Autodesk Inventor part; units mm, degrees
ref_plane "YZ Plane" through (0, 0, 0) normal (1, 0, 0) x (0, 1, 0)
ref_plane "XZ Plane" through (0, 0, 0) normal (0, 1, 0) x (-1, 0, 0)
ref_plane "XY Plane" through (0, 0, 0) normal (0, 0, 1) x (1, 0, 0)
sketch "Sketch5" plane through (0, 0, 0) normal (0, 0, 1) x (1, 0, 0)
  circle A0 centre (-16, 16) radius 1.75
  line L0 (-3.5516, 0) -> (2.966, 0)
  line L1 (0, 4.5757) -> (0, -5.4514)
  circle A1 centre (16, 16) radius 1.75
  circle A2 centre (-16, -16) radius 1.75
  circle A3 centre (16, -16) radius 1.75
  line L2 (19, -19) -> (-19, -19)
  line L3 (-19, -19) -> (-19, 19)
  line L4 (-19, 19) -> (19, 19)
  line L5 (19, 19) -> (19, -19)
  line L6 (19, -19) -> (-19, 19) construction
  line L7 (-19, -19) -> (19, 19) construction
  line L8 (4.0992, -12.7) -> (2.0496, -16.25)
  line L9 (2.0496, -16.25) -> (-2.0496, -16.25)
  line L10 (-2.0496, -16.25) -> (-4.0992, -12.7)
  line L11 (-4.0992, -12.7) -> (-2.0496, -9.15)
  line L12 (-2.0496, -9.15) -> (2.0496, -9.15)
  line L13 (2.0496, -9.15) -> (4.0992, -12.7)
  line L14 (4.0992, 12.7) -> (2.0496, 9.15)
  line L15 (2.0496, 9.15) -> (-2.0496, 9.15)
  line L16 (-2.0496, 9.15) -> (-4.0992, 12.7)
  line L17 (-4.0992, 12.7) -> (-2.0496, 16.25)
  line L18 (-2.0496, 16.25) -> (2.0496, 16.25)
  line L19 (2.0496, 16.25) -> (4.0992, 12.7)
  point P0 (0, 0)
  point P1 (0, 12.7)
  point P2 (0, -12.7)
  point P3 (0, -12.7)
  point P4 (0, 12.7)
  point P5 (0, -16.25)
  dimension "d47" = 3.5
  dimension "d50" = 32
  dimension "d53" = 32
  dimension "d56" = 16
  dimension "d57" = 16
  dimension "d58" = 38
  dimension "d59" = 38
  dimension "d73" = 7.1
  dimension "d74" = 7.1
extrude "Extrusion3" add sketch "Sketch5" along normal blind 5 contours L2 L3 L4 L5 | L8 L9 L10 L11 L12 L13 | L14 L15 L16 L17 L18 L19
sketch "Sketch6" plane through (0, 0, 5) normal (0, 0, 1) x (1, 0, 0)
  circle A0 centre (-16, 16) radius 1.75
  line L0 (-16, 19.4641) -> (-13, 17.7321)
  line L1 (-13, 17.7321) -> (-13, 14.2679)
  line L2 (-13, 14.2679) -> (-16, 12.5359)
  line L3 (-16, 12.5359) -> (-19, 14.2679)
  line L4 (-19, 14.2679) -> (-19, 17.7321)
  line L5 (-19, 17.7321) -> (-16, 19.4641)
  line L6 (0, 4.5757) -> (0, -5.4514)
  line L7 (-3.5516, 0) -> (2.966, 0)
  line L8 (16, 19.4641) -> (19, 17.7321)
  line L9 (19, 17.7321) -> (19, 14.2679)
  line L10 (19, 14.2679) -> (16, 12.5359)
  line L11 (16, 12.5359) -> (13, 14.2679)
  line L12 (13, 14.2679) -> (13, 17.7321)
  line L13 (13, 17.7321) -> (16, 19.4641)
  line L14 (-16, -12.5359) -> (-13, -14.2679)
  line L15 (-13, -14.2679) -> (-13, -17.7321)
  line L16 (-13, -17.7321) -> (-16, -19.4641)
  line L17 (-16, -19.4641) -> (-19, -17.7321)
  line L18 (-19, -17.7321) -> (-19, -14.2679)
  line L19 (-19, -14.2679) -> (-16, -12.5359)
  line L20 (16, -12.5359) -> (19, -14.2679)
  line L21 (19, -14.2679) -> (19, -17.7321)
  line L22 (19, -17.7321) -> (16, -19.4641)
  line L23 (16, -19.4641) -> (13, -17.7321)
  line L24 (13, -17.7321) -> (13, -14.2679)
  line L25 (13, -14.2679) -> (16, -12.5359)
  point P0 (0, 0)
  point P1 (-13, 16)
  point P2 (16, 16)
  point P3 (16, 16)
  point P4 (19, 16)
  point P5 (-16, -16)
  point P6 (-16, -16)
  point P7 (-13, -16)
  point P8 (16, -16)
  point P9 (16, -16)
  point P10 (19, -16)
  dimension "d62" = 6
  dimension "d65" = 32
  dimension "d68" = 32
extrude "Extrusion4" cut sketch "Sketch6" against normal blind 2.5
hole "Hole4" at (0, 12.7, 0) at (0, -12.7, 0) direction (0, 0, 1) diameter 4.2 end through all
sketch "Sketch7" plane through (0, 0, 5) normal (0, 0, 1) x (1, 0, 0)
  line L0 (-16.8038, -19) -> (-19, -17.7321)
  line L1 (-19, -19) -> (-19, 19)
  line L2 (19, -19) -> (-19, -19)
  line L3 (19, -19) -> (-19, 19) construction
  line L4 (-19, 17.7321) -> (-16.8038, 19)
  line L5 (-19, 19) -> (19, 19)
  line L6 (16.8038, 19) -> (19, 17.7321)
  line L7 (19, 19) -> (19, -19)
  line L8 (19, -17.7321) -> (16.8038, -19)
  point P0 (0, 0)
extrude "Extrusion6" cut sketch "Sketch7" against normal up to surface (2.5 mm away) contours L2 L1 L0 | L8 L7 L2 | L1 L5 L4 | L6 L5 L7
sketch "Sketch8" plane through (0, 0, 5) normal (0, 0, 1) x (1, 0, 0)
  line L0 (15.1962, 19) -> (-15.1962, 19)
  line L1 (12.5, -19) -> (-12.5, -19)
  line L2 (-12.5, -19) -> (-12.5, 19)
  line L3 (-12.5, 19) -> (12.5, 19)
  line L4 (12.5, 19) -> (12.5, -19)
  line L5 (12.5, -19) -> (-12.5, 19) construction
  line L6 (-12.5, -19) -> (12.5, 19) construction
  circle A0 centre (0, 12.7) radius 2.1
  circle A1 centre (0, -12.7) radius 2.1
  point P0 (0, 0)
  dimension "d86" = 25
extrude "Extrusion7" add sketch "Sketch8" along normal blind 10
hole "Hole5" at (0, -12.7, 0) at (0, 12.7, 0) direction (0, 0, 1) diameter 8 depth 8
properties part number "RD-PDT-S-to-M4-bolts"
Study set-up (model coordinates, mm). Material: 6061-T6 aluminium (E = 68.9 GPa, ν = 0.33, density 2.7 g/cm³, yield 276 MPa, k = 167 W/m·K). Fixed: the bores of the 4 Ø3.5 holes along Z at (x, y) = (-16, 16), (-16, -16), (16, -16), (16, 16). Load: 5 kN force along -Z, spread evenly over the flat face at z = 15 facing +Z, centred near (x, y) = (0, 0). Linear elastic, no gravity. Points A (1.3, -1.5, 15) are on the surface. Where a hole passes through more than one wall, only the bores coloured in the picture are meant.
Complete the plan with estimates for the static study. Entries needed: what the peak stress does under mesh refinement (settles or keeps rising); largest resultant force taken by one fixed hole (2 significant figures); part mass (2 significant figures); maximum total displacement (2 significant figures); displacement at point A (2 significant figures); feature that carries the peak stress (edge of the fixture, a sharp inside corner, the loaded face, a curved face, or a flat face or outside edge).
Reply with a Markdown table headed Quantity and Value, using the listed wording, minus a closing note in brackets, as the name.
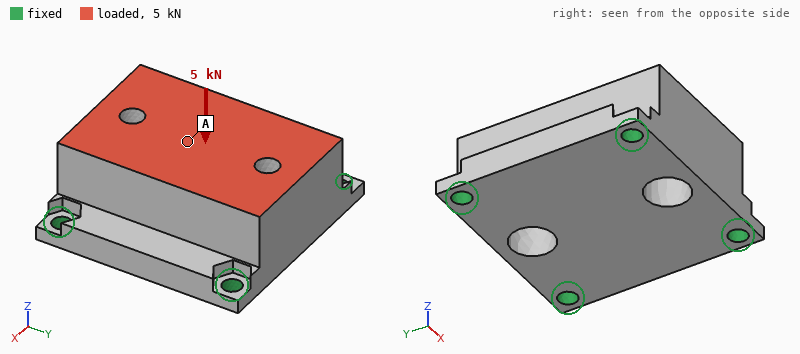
| Quantity | Value |
|---|---|
| what the peak stress does under mesh refinement | keeps rising |
| largest resultant force taken by one fixed hole | 1.5 kN |
| part mass | 41 g |
| maximum total displacement | 16 µm |
| displacement at point A | 16 µm |
| feature that carries the peak stress | edge of the fixture |
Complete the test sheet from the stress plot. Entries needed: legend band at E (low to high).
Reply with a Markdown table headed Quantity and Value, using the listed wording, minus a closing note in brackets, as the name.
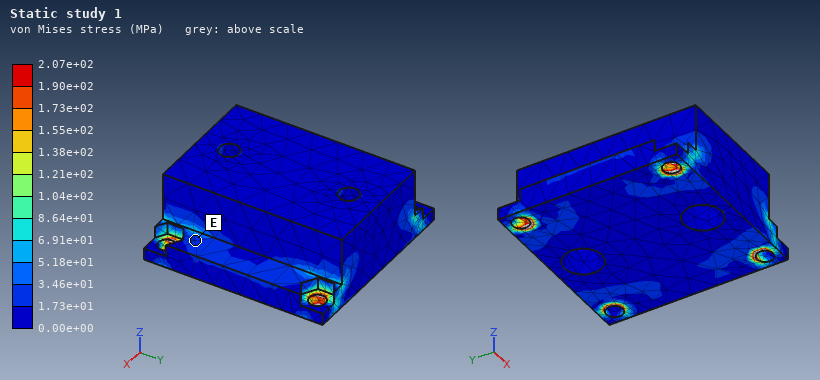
| Quantity | Value |
|---|---|
| legend band at E | 1.73e+01 to 3.46e+01 MPa |
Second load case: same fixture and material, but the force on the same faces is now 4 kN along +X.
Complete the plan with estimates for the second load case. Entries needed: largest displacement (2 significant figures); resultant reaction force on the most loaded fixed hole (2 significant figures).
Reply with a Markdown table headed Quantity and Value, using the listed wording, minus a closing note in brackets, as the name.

| Quantity | Value |
|---|---|
| largest displacement | 17 µm |
| resultant reaction force on the most loaded fixed hole | 1.4 kN |
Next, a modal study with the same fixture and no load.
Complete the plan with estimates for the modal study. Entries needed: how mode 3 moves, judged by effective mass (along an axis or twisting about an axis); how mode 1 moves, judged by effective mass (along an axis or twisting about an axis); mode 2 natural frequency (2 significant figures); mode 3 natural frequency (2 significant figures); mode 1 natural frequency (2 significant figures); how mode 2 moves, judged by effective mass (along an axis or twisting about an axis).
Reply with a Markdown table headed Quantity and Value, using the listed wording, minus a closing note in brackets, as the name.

| Quantity | Value |
|---|---|
| how mode 3 moves, judged by effective mass | along X |
| how mode 1 moves, judged by effective mass | along Z |
| mode 2 natural frequency | 17 kHz |
| mode 3 natural frequency | 19 kHz |
| mode 1 natural frequency | 15 kHz |
| how mode 2 moves, judged by effective mass | along Y |
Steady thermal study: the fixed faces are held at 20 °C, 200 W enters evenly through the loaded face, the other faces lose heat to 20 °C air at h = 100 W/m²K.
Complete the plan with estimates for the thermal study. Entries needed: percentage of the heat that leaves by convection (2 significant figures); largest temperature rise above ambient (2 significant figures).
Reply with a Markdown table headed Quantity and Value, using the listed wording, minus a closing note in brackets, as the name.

| Quantity | Value |
|---|---|
| percentage of the heat that leaves by convection | 9.4 % |
| largest temperature rise above ambient | 62 K |
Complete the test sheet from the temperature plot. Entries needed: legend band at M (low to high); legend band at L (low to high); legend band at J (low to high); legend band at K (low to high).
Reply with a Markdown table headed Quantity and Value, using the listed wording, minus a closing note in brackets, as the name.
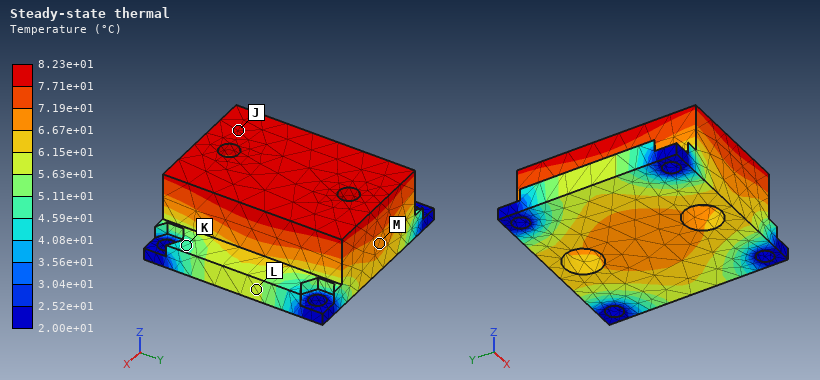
| Quantity | Value |
|---|---|
| legend band at M | 6.67e+01 to 7.19e+01 °C |
| legend band at L | 5.63e+01 to 6.15e+01 °C |
| legend band at J | 7.71e+01 to 8.23e+01 °C |
| legend band at K | 4.59e+01 to 5.11e+01 °C |
